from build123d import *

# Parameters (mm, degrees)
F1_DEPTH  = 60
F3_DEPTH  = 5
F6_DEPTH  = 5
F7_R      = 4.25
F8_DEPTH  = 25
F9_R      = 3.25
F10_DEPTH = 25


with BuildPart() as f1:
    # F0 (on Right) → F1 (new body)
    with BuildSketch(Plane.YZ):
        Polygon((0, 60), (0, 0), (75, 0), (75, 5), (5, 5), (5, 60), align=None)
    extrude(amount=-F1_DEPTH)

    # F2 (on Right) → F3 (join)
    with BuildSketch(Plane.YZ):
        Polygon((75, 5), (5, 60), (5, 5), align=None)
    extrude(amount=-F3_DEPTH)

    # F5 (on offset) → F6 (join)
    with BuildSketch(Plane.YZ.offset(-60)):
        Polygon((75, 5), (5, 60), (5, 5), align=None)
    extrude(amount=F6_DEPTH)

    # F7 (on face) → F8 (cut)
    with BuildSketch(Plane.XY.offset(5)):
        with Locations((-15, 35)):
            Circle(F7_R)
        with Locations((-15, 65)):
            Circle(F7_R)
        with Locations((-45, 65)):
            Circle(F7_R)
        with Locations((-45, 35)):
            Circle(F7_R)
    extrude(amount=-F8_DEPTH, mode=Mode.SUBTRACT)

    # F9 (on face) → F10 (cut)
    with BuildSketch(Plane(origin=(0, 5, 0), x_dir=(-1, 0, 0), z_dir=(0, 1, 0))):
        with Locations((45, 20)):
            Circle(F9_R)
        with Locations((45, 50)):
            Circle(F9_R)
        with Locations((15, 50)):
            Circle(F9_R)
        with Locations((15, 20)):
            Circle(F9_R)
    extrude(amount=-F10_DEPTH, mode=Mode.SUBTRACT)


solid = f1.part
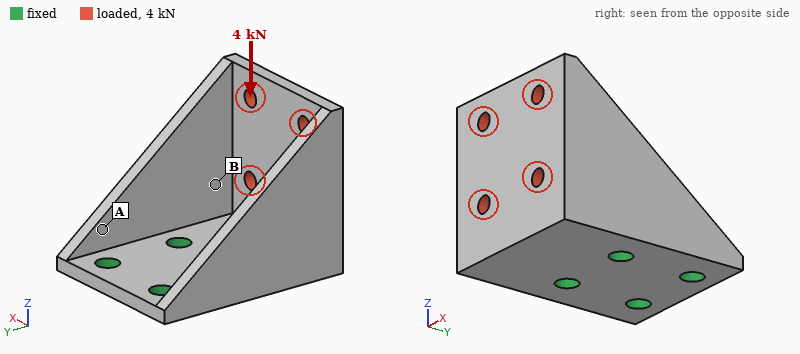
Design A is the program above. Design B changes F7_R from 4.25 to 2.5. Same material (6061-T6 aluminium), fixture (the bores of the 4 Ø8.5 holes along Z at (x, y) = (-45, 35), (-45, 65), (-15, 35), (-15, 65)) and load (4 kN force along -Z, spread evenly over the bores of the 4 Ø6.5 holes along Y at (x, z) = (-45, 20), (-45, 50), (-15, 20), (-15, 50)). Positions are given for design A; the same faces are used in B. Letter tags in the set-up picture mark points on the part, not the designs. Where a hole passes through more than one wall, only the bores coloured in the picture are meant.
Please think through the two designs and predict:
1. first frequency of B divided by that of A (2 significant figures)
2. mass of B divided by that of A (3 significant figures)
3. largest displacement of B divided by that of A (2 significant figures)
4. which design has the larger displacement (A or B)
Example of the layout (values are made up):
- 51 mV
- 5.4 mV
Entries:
- 0.87
- 1.01
- 1.4
- B
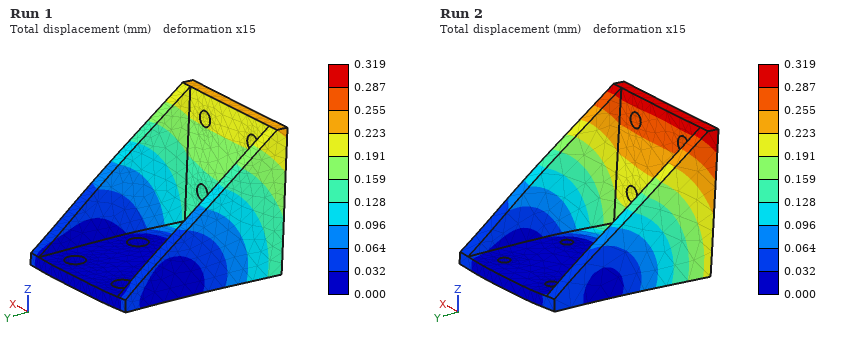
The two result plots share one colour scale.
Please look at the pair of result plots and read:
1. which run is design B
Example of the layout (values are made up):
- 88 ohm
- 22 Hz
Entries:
- Run 2
